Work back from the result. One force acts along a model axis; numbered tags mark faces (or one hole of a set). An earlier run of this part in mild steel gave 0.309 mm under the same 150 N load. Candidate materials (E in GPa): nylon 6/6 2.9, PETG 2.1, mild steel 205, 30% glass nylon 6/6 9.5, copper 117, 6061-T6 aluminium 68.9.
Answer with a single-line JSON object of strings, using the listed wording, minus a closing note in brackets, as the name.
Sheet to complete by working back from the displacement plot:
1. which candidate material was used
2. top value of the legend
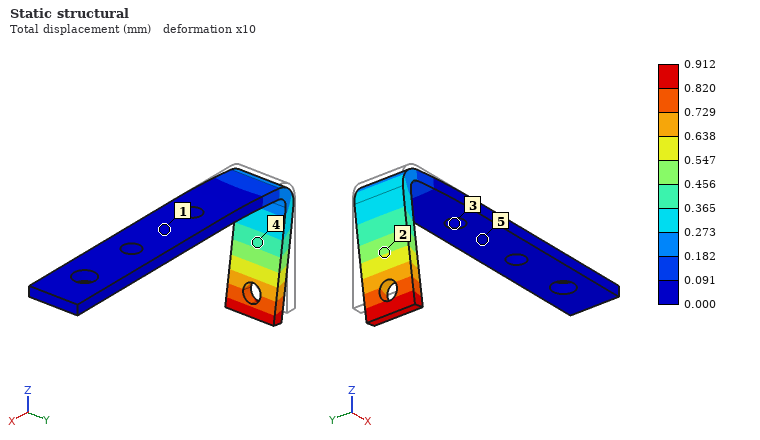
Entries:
{"which candidate material was used": "6061-T6 aluminium", "top value of the legend": "0.912 mm"}
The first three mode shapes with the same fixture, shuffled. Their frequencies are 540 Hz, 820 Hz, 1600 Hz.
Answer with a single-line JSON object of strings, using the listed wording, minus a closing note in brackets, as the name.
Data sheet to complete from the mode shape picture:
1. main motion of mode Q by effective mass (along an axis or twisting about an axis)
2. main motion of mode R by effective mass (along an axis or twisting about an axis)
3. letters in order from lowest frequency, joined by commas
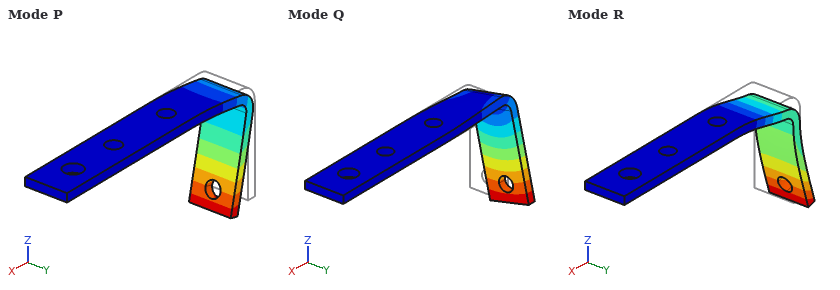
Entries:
{"main motion of mode Q by effective mass": "along Y", "main motion of mode R by effective mass": "along Z", "letters in order from lowest frequency, joined by commas": "P, Q, R"}
